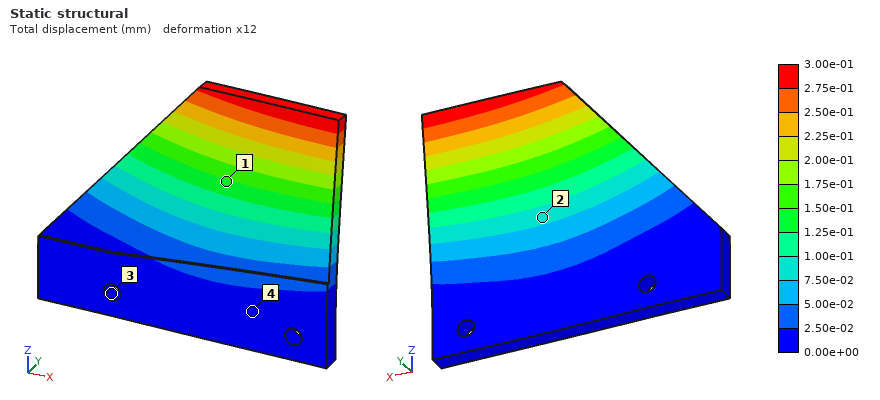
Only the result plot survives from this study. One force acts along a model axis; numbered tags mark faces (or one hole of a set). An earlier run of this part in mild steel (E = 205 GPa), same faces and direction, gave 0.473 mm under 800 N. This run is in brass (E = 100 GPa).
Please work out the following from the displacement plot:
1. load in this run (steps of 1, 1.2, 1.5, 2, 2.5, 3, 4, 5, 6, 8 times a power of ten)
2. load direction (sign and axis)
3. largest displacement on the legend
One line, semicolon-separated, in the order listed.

250 N; +Y; 3.00e-01 mm
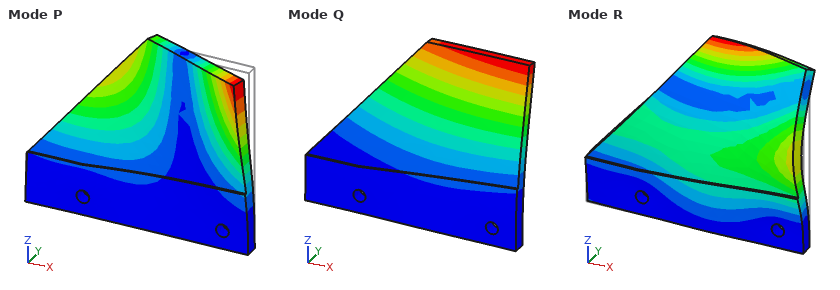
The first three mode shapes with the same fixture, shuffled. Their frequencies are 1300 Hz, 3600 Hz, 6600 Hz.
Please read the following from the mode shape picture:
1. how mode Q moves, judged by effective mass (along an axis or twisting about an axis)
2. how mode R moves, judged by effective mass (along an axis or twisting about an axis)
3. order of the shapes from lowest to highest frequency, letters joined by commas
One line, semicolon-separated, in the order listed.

along Y; along Y; Q, P, R
